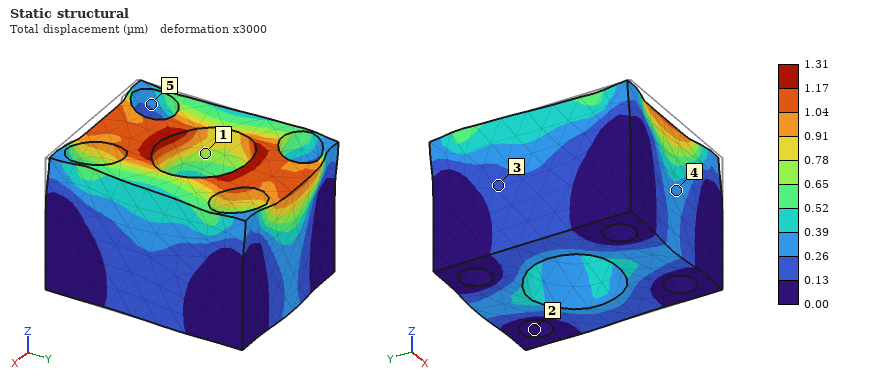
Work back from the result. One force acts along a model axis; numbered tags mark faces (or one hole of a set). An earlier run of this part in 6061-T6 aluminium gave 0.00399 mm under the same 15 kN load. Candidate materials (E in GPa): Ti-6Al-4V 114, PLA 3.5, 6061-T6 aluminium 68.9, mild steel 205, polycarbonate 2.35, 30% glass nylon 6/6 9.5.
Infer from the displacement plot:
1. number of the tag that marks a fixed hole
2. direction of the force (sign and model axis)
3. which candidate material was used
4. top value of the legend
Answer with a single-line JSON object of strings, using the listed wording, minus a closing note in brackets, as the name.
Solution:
{"number of the tag that marks a fixed hole": "2", "direction of the force": "+Y", "which candidate material was used": "mild steel", "top value of the legend": "1.31 µm"}
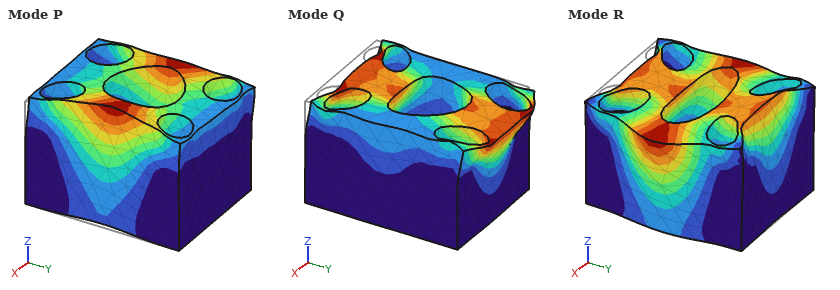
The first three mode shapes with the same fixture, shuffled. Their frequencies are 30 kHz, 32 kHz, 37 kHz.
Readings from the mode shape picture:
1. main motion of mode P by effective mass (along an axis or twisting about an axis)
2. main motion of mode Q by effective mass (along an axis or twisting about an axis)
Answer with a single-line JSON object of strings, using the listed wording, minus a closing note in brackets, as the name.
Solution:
{"main motion of mode P by effective mass": "along X", "main motion of mode Q by effective mass": "along Y"}
